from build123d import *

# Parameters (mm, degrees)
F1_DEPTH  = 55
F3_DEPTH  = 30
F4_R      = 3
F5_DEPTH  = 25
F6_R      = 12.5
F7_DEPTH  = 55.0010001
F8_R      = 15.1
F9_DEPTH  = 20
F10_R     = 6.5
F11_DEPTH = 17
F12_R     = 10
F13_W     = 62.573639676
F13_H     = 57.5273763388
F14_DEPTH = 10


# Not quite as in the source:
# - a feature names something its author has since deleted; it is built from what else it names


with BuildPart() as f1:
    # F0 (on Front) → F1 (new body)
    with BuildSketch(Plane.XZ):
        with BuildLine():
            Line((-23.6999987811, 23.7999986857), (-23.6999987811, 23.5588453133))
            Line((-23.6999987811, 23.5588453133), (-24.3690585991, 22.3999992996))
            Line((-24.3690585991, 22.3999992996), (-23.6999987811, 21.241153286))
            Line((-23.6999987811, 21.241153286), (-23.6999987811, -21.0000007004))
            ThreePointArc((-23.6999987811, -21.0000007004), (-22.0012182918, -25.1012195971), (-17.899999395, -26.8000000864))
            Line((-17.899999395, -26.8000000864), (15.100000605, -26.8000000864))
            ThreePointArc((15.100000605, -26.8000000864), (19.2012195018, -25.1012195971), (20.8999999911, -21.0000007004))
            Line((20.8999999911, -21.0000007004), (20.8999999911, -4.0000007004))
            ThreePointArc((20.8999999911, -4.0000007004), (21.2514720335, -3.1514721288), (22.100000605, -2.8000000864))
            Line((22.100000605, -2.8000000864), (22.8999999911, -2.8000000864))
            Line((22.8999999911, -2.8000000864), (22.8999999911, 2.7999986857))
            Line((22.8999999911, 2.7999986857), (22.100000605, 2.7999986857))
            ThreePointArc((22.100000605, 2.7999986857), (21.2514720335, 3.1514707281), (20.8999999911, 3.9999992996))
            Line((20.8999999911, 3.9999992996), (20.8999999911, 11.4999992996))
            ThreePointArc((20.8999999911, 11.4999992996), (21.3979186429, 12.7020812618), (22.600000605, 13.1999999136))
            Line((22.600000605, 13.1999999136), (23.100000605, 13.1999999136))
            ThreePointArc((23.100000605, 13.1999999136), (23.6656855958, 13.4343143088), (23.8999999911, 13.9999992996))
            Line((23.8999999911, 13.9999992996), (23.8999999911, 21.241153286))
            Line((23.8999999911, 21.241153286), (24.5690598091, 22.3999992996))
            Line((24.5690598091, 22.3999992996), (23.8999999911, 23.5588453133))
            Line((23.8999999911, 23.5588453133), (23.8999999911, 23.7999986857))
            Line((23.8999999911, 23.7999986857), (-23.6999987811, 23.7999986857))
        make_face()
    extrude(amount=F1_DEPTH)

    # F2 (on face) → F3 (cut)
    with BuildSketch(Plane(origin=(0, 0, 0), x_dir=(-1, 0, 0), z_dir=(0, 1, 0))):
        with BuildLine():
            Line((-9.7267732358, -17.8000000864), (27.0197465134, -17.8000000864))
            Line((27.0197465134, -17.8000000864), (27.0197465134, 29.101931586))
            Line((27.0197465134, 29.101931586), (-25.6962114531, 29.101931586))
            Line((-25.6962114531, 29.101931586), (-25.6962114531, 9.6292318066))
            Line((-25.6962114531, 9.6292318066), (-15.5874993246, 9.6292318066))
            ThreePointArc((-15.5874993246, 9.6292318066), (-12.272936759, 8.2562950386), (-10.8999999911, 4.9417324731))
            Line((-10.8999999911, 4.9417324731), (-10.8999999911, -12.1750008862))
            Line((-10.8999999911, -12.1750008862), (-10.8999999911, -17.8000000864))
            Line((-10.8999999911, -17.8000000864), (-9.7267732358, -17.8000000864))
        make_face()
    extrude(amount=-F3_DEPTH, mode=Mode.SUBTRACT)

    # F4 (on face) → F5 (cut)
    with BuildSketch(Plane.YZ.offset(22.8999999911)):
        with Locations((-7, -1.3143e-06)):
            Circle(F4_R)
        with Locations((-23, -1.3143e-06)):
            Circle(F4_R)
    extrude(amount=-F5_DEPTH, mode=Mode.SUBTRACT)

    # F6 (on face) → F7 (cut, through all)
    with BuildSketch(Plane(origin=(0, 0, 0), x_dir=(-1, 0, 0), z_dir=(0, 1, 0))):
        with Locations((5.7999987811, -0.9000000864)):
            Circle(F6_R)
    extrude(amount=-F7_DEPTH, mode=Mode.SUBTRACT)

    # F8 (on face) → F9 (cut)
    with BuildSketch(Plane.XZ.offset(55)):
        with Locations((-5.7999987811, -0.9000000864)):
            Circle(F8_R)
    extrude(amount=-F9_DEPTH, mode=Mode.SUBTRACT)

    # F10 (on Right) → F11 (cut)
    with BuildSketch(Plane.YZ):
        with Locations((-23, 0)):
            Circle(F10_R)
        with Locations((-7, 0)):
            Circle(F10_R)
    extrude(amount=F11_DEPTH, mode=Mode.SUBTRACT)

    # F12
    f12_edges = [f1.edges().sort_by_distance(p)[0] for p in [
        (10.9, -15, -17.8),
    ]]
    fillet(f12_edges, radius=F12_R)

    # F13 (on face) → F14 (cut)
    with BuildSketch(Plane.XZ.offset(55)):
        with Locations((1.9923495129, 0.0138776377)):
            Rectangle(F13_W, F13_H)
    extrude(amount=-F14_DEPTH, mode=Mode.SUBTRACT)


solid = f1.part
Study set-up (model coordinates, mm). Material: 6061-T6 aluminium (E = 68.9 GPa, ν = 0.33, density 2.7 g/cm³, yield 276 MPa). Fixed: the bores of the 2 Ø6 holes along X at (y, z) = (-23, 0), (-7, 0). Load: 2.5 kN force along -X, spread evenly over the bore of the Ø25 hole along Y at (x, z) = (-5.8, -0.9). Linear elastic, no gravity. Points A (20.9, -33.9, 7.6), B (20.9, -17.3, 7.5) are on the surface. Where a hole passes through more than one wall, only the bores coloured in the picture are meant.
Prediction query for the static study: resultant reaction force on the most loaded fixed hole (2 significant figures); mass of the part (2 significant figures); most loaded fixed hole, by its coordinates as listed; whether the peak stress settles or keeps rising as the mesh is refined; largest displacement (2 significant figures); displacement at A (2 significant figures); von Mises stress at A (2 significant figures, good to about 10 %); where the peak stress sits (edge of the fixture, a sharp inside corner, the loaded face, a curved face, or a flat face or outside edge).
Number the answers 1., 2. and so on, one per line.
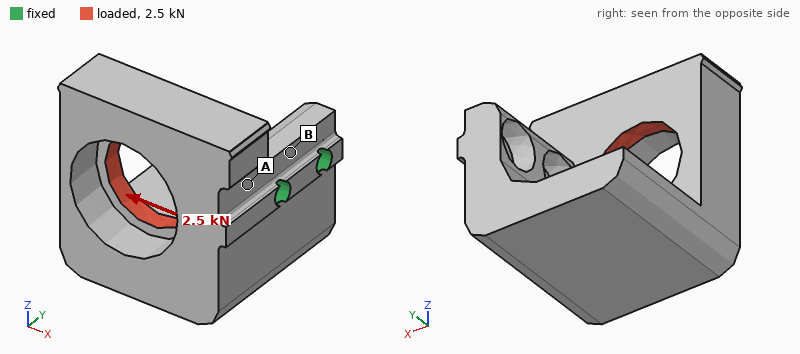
1. 3.2 kN
2. 120 g
3. (-23, 0)
4. keeps rising
5. 62 µm
6. 20 µm
7. 18 MPa
8. edge of the fixture
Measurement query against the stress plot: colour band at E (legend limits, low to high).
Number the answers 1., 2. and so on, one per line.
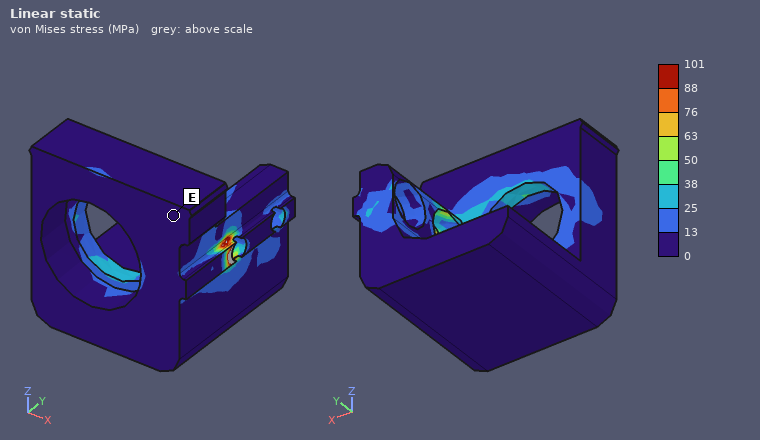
1. 0 to 13 MPa
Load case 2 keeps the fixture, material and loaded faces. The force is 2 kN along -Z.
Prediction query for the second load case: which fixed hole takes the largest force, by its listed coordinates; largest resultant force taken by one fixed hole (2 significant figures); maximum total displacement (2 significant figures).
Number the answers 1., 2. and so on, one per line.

1. (-23, 0)
2. 2.6 kN
3. 0.33 mm
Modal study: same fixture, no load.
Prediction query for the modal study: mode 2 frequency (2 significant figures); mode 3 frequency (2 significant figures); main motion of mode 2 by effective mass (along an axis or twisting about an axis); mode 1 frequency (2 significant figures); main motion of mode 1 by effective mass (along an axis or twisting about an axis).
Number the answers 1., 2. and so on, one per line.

1. 2600 Hz
2. 4800 Hz
3. along Y
4. 1500 Hz
5. along Z
